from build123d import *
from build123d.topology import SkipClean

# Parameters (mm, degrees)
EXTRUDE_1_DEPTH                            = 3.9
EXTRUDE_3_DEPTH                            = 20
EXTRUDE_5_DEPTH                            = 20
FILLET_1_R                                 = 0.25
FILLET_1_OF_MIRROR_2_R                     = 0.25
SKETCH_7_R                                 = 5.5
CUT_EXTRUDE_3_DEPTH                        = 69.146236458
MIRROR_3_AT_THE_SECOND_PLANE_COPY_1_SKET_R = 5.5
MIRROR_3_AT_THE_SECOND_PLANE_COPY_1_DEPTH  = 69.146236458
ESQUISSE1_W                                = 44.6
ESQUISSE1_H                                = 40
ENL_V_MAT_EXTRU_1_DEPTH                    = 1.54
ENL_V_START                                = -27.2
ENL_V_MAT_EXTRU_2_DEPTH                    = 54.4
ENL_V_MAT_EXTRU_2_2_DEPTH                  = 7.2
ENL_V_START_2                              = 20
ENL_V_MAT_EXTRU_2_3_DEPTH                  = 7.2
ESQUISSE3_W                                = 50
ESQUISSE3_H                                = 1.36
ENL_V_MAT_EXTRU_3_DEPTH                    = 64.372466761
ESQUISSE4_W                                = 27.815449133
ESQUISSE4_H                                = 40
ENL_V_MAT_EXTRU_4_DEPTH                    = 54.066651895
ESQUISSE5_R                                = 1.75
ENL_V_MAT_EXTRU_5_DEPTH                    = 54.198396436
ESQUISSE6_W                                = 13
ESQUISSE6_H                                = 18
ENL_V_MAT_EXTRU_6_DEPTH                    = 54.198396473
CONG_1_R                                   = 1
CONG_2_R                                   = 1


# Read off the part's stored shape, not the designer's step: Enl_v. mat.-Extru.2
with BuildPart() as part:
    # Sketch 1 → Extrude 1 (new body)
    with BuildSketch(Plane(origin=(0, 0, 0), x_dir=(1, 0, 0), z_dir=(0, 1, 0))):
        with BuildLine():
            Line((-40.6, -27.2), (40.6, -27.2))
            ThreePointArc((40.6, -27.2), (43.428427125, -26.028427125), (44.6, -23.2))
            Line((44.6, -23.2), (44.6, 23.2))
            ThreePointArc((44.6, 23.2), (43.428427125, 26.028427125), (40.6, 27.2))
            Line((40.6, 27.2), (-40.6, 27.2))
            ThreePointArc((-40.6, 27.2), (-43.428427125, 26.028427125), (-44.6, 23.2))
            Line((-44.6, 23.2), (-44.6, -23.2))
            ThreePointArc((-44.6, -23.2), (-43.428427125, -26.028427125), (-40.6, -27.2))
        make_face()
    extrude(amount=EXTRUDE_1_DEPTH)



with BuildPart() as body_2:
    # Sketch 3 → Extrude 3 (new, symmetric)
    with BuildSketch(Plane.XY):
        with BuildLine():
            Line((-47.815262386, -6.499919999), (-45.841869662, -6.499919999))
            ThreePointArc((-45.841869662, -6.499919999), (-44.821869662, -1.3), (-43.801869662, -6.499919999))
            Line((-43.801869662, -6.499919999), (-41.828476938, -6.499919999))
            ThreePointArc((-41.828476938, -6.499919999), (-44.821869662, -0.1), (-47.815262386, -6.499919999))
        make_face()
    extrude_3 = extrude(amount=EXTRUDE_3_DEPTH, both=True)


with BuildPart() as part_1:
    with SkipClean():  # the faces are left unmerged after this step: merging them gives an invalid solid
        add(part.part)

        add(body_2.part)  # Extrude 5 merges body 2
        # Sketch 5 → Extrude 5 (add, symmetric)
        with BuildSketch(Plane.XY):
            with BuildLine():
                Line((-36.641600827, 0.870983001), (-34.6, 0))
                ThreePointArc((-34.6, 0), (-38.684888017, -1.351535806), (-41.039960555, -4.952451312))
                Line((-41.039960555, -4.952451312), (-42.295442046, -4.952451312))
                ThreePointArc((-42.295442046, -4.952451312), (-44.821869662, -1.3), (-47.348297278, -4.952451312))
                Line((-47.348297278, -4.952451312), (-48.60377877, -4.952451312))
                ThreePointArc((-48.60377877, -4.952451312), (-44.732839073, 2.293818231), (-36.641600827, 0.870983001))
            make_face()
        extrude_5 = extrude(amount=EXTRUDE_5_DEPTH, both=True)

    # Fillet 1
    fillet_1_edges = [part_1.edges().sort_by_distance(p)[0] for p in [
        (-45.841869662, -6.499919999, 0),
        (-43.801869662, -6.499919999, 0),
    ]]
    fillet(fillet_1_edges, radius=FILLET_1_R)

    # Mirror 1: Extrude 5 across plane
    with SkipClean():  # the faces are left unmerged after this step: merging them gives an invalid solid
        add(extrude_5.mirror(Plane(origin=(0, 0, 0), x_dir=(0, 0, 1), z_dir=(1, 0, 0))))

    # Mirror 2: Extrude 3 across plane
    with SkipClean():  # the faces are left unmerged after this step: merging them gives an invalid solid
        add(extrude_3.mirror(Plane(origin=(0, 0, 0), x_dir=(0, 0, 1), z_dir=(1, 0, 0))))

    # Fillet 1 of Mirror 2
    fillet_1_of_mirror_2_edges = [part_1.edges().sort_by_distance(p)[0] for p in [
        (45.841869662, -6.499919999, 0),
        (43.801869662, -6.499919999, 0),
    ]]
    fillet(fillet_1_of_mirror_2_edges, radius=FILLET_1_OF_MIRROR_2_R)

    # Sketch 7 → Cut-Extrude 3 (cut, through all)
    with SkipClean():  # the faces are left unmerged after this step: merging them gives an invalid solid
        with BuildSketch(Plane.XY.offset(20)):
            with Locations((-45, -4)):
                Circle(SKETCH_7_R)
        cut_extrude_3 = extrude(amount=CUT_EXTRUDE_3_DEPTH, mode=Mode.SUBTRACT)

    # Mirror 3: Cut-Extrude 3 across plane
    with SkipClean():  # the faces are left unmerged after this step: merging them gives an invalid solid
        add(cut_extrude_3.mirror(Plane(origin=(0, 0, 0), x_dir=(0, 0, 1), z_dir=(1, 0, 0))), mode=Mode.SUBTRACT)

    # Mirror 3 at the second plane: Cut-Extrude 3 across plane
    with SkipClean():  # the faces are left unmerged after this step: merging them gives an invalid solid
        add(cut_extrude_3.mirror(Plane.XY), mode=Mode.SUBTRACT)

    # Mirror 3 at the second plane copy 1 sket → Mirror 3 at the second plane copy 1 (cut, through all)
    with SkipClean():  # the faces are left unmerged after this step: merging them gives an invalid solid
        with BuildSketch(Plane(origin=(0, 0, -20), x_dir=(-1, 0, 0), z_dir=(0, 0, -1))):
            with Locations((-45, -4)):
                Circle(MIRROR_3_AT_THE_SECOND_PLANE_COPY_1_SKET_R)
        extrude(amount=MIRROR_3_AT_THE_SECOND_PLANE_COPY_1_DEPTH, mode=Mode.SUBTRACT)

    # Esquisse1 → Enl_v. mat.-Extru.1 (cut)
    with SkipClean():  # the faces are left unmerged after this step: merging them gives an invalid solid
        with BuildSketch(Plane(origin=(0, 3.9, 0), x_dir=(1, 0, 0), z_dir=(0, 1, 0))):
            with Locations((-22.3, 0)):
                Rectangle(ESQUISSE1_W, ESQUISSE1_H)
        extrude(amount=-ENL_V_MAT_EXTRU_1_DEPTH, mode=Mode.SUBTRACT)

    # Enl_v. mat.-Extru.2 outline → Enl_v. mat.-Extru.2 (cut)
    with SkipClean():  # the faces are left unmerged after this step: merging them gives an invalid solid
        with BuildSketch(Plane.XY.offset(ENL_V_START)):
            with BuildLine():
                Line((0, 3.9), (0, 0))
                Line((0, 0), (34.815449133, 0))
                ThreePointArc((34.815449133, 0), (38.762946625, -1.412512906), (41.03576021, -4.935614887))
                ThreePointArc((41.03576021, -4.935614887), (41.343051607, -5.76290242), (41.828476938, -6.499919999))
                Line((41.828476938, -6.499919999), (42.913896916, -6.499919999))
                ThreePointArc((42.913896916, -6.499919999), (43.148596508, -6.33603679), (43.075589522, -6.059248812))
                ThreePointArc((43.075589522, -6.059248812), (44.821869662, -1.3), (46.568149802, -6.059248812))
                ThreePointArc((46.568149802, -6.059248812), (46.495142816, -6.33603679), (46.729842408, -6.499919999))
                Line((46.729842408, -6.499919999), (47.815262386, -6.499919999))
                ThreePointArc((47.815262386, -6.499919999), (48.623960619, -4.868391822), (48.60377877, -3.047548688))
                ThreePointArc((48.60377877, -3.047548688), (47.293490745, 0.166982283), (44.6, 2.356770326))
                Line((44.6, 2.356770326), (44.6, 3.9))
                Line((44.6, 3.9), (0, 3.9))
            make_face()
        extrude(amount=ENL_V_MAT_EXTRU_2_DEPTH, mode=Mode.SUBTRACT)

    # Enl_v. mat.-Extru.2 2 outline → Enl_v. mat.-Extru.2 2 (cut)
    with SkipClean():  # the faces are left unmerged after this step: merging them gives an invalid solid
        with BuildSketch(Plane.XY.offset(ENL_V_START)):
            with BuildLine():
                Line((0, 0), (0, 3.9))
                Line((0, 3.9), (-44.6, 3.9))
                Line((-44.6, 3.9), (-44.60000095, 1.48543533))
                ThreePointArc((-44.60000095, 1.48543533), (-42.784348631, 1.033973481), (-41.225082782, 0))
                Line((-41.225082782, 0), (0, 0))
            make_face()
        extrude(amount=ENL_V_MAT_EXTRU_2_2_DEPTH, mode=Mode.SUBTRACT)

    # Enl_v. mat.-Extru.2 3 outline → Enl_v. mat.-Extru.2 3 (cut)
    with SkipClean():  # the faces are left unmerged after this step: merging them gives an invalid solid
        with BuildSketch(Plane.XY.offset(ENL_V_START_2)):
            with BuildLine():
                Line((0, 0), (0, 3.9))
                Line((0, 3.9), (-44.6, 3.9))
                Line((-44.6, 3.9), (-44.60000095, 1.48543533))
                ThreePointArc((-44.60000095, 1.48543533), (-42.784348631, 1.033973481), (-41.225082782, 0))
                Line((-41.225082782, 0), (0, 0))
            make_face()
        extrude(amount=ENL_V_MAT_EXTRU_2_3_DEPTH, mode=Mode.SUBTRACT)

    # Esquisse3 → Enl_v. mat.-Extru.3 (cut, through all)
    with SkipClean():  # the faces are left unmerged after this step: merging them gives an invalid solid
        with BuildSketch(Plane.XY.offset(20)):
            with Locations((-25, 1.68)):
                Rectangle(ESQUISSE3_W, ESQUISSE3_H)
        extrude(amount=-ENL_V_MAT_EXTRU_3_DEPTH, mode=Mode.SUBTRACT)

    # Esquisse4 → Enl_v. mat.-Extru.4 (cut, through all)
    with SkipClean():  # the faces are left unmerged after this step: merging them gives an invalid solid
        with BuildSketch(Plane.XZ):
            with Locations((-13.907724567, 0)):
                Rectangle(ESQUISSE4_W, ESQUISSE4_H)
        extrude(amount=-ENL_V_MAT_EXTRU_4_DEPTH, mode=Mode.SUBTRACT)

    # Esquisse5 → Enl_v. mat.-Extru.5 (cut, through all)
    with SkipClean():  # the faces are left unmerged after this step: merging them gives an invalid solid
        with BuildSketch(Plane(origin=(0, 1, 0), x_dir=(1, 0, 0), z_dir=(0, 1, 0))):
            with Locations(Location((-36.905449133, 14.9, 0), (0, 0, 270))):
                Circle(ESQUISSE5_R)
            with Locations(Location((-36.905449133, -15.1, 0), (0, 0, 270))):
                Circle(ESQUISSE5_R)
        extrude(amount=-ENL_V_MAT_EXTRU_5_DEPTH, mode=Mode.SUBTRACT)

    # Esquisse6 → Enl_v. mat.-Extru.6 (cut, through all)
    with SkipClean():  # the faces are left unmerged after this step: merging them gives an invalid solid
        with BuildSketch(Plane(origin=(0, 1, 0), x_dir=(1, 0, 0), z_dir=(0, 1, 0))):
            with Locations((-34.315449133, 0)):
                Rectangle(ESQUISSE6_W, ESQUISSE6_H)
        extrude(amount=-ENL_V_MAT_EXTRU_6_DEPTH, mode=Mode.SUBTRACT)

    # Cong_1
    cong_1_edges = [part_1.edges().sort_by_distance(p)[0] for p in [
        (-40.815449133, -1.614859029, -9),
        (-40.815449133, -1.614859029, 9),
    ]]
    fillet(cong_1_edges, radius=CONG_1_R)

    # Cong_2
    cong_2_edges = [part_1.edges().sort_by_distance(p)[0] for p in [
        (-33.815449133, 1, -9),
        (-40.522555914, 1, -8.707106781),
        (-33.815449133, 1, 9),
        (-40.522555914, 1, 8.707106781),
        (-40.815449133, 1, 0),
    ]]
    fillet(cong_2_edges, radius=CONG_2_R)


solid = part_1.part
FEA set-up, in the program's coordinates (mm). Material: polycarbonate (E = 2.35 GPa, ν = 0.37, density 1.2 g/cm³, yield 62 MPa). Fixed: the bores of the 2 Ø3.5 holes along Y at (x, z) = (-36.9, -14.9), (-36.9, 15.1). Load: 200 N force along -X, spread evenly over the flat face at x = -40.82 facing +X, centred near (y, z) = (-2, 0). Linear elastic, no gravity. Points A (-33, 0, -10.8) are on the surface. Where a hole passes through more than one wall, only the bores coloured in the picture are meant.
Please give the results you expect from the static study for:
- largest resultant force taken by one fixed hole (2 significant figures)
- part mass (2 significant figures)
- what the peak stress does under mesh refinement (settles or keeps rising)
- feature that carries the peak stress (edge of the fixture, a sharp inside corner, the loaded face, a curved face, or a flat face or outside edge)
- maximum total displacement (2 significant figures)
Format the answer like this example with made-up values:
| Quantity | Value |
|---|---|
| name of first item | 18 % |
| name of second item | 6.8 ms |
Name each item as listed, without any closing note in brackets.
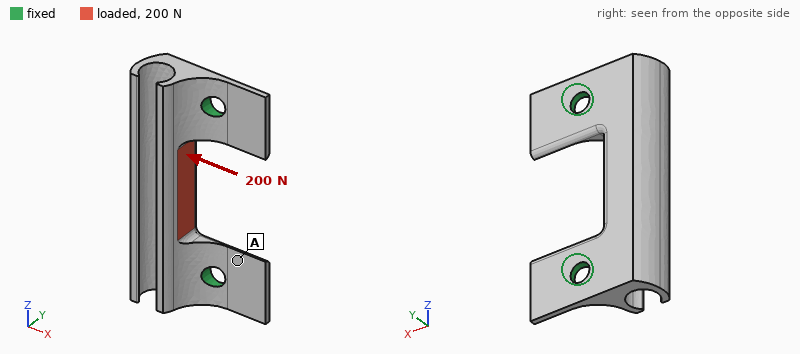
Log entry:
| Quantity | Value |
|---|---|
| largest resultant force taken by one fixed hole | 130 N |
| part mass | 2.0 g |
| what the peak stress does under mesh refinement | keeps rising |
| feature that carries the peak stress | edge of the fixture |
| maximum total displacement | 0.47 mm |
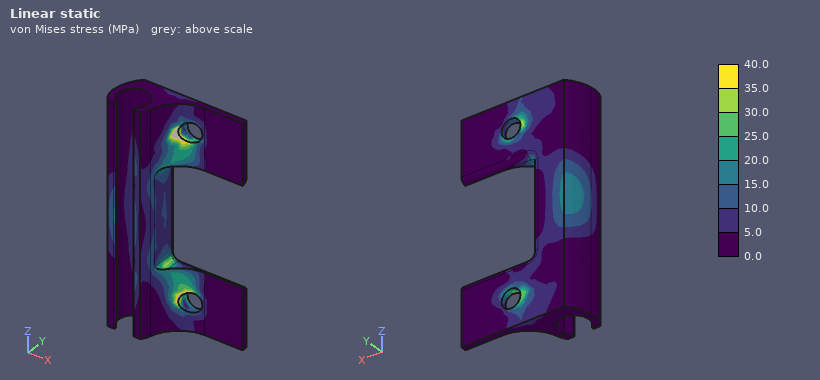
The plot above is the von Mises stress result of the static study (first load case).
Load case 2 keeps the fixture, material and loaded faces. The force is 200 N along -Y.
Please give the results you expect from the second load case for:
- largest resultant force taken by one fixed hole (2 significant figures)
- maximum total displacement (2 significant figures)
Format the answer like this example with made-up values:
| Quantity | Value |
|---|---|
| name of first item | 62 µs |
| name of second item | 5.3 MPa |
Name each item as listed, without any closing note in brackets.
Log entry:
| Quantity | Value |
|---|---|
| largest resultant force taken by one fixed hole | 110 N |
| maximum total displacement | 0.38 mm |
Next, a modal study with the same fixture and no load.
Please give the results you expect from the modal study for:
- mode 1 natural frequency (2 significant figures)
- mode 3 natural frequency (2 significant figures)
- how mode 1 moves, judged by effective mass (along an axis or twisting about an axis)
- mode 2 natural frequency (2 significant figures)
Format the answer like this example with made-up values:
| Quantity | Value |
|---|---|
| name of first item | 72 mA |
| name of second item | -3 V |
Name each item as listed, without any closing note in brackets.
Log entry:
| Quantity | Value |
|---|---|
| mode 1 natural frequency | 2400 Hz |
| mode 3 natural frequency | 3700 Hz |
| how mode 1 moves, judged by effective mass | along Y |
| mode 2 natural frequency | 3700 Hz |
